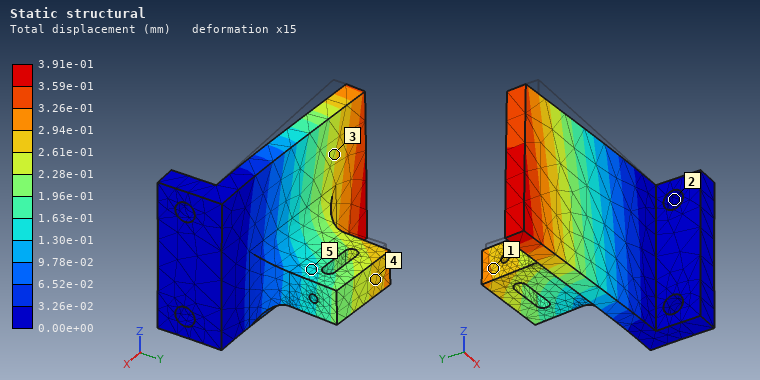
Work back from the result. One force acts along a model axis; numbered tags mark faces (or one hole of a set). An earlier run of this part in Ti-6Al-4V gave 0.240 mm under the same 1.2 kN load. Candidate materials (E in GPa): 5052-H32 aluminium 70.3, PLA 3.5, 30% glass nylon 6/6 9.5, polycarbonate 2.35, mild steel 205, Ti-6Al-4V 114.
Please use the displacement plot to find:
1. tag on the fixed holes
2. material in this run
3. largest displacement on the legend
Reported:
2
5052-H32 aluminium
3.91e-01 mm
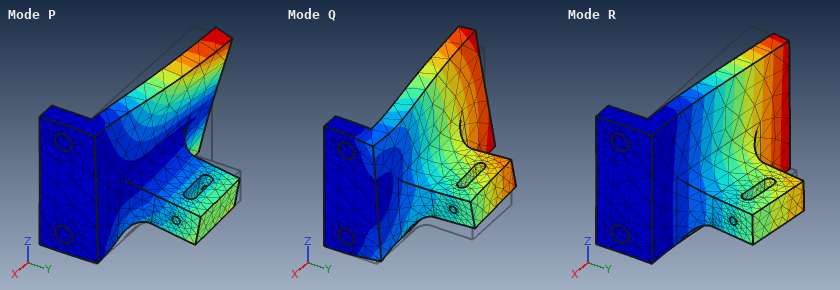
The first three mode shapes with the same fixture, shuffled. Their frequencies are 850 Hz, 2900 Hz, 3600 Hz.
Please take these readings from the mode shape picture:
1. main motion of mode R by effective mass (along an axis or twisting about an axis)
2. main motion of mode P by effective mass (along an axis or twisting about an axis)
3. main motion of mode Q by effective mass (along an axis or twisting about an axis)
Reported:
along Y
twisting about X
along Z
